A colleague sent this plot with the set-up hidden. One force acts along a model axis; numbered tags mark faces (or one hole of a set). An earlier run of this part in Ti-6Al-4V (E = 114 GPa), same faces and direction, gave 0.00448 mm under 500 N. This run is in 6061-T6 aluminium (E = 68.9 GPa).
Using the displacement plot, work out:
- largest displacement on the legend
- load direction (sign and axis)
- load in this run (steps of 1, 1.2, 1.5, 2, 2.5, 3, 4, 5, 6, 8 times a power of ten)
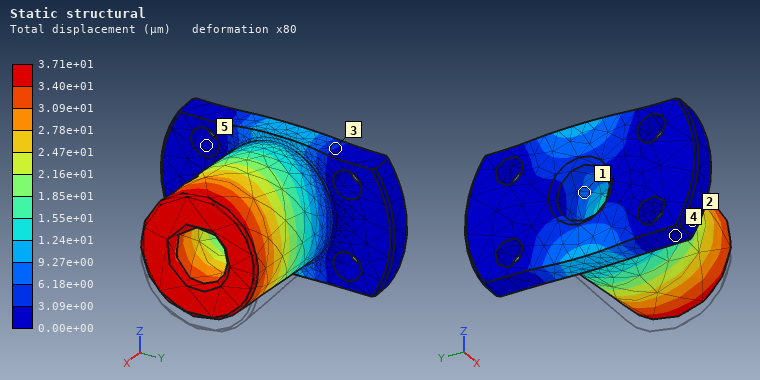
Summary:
3.71e+01 µm
+Z
2.5 kN
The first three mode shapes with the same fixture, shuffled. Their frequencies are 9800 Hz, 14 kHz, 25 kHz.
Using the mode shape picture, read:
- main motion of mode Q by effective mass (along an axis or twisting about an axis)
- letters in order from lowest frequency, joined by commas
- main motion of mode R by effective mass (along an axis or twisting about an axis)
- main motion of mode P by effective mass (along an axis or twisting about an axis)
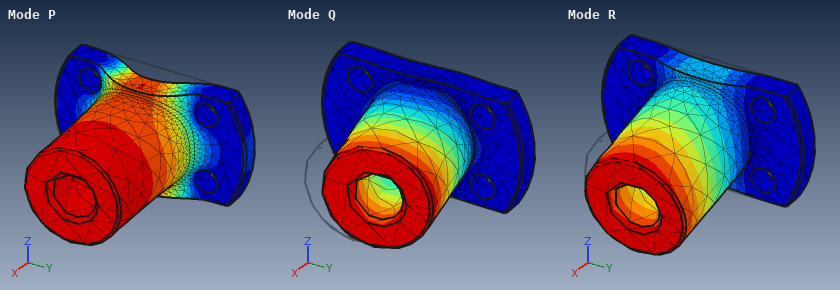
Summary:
along Y
R, Q, P
along Z
along X
